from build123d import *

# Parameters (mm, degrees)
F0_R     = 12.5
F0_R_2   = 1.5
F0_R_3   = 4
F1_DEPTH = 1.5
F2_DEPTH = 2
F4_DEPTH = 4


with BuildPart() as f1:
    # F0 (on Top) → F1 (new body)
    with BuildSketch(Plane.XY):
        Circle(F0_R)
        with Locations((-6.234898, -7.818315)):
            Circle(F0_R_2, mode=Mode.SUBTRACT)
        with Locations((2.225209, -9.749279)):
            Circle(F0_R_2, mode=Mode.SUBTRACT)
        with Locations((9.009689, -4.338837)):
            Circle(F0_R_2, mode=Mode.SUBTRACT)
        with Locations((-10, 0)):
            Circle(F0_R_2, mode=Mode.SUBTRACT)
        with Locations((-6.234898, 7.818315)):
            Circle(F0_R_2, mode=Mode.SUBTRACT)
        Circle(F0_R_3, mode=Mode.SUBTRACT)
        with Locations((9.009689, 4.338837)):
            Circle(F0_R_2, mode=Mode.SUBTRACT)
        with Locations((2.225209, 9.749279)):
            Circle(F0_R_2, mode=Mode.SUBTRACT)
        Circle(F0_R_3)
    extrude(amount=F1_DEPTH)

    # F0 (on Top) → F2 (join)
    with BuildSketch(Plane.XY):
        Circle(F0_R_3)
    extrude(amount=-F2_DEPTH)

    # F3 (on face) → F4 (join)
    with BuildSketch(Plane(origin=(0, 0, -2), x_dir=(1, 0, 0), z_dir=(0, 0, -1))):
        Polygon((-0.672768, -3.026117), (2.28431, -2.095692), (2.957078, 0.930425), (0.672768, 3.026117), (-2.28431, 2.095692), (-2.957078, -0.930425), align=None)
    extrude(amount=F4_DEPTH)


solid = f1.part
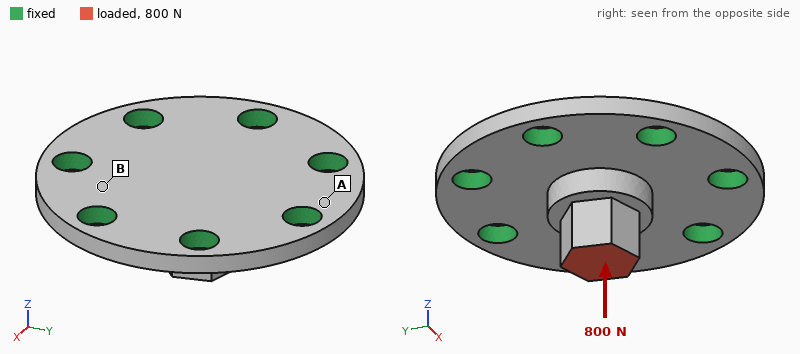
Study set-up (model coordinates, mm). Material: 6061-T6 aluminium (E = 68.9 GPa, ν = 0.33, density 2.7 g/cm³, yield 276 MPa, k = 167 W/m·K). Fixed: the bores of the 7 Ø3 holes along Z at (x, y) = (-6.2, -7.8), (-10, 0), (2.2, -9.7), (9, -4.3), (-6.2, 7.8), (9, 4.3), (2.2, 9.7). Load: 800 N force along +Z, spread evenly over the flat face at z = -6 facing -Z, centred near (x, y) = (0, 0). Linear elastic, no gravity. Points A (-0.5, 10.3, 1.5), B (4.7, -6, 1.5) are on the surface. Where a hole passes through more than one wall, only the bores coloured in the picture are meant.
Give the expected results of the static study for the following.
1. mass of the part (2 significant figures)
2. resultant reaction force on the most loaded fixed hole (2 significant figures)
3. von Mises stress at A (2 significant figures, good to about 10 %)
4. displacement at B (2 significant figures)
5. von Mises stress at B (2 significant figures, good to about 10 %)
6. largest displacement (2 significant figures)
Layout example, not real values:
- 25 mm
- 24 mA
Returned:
- 2.3 g
- 130 N
- 24 MPa
- 4.7 µm
- 58 MPa
- 23 µm
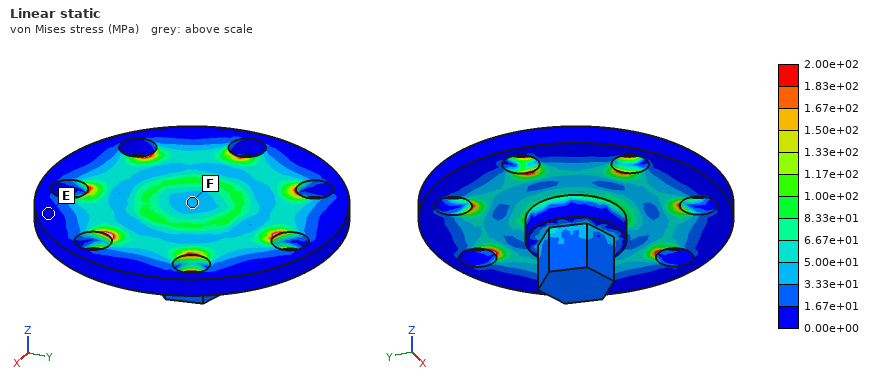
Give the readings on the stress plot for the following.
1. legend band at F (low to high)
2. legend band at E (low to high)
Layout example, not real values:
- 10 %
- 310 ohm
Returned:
- 3.33e+01 to 5.00e+01 MPa
- 0.00e+00 to 1.67e+01 MPa
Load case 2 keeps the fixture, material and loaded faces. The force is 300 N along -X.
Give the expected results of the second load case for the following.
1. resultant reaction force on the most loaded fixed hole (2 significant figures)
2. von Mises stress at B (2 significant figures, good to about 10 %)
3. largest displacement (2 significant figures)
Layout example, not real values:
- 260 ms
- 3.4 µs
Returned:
- 110 N
- 21 MPa
- 24 µm
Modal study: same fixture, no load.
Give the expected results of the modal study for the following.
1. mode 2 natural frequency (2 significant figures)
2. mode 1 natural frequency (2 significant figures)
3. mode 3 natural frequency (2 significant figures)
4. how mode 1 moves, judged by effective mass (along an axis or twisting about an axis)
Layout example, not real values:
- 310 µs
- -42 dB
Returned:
- 41 kHz
- 33 kHz
- 41 kHz
- along Z
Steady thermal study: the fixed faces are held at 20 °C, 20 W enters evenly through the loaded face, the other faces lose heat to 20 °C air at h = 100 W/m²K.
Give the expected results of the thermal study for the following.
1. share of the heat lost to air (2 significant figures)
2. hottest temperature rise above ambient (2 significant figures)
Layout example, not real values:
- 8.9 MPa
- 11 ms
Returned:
- 3.0 %
- 40 K
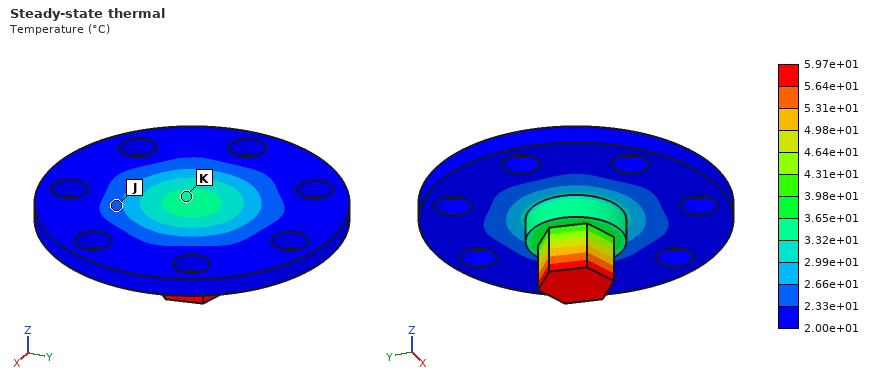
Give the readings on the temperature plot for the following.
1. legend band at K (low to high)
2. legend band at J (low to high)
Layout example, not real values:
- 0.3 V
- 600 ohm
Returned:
- 3.32e+01 to 3.65e+01 °C
- 2.33e+01 to 2.66e+01 °C
